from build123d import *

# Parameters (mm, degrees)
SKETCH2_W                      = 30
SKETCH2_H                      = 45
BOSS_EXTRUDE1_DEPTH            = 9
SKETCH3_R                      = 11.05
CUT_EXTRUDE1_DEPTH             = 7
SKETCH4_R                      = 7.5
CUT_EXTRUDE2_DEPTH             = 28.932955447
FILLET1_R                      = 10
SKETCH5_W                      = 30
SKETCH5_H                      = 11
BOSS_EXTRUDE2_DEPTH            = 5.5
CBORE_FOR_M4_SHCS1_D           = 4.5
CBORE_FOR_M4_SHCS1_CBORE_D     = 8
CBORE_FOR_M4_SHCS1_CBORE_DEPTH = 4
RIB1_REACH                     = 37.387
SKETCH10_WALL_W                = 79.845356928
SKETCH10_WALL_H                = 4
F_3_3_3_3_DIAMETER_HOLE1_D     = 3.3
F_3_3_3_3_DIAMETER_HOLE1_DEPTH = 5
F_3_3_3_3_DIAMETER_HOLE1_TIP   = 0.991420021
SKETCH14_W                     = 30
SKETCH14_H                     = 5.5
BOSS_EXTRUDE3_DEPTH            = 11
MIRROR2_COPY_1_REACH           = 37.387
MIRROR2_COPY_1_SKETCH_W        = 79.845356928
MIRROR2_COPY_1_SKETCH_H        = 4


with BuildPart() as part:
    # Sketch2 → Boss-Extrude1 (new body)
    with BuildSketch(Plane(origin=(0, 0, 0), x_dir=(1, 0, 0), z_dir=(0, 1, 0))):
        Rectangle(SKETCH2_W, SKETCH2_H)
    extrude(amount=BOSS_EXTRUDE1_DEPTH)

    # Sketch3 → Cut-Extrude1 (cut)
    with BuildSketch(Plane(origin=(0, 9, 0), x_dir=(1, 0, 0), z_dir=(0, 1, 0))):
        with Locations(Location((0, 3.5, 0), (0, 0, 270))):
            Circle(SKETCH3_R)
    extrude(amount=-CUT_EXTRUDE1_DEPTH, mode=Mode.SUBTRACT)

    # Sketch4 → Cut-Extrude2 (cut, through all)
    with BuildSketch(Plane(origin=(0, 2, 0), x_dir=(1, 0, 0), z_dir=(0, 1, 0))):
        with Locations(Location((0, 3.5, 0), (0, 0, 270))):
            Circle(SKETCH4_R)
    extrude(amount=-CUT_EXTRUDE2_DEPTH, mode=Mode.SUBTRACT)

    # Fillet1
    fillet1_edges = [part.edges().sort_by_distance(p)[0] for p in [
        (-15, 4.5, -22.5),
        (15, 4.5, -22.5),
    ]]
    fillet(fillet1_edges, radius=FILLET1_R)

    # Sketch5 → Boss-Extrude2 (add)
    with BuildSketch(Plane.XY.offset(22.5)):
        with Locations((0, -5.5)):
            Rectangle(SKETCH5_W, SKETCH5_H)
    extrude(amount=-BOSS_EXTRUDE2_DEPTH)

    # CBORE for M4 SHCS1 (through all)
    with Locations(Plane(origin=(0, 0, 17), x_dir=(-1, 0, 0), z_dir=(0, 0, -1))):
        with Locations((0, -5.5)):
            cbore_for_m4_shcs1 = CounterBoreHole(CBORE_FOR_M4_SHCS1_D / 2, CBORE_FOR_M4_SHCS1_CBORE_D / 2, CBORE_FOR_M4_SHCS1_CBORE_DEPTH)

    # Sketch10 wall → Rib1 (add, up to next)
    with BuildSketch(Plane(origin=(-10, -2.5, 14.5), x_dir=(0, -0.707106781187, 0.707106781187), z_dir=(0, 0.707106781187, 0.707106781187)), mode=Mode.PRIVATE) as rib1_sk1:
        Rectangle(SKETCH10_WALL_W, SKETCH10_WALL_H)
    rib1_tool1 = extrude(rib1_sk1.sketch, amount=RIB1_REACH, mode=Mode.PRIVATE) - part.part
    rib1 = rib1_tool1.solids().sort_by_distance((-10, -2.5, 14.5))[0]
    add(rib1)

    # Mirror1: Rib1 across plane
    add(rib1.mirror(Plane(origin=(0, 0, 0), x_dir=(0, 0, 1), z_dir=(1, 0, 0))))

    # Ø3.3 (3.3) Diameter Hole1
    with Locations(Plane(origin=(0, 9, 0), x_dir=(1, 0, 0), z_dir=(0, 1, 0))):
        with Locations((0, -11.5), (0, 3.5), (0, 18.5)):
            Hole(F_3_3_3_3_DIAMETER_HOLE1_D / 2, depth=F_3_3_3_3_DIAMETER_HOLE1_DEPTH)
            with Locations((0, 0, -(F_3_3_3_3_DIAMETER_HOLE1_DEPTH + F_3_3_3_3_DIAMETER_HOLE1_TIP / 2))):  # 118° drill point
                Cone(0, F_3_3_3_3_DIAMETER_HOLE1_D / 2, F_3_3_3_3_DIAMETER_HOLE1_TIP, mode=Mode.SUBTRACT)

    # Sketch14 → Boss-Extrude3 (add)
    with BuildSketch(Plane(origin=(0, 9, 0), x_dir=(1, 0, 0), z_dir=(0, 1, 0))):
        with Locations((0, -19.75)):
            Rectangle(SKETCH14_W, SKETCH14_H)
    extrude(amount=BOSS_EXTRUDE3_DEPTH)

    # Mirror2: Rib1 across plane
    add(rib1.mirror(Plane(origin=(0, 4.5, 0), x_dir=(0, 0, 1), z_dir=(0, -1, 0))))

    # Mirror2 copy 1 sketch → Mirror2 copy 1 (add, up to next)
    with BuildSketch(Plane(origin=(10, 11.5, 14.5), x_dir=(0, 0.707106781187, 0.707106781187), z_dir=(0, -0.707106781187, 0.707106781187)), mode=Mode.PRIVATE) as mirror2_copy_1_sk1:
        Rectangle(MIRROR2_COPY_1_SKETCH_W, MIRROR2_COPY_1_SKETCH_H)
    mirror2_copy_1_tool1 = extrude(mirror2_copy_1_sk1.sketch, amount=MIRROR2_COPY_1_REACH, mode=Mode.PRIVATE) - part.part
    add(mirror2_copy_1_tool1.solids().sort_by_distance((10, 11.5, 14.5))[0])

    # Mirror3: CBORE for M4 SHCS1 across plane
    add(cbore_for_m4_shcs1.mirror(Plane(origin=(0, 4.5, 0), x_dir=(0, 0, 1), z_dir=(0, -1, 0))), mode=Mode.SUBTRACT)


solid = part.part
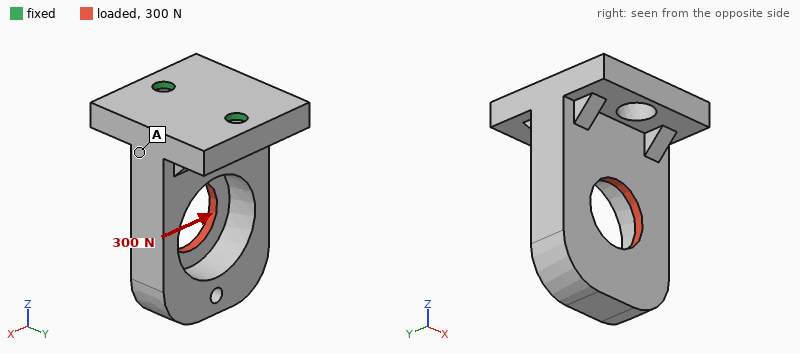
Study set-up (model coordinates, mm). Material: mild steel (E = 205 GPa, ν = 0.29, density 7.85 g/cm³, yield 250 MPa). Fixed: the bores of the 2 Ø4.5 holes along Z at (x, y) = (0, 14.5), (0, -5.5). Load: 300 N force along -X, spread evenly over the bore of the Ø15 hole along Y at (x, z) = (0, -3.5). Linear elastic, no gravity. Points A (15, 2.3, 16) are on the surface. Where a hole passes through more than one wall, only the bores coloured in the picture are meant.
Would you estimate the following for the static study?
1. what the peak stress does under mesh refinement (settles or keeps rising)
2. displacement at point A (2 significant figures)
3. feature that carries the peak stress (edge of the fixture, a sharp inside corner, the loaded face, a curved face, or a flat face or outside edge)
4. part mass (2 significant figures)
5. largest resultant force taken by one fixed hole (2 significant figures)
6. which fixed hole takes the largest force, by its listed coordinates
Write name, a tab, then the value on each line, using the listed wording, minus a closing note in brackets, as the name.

what the peak stress does under mesh refinement	keeps rising
displacement at point A	25 µm
feature that carries the peak stress	edge of the fixture
part mass	94 g
largest resultant force taken by one fixed hole	200 N
which fixed hole takes the largest force, by its listed coordinates	(0, -5.5)
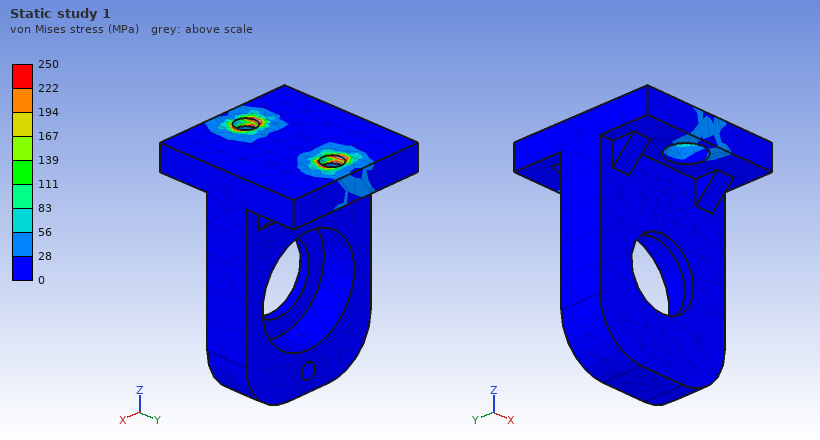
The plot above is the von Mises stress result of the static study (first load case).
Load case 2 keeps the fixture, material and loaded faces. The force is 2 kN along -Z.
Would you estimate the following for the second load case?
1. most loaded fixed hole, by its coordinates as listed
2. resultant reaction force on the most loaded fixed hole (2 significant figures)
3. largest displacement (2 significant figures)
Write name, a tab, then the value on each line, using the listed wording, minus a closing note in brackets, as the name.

most loaded fixed hole, by its coordinates as listed	(0, -5.5)
resultant reaction force on the most loaded fixed hole	1.4 kN
largest displacement	23 µm
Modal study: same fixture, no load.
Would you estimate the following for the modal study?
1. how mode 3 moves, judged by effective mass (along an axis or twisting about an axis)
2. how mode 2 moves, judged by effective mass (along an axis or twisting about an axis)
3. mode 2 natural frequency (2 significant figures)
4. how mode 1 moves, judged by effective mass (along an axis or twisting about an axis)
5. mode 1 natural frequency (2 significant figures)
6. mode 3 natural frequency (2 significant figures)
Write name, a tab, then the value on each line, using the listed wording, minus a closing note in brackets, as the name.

how mode 3 moves, judged by effective mass	twisting about Z
how mode 2 moves, judged by effective mass	along Y
mode 2 natural frequency	3500 Hz
how mode 1 moves, judged by effective mass	along X
mode 1 natural frequency	1600 Hz
mode 3 natural frequency	9200 Hz
